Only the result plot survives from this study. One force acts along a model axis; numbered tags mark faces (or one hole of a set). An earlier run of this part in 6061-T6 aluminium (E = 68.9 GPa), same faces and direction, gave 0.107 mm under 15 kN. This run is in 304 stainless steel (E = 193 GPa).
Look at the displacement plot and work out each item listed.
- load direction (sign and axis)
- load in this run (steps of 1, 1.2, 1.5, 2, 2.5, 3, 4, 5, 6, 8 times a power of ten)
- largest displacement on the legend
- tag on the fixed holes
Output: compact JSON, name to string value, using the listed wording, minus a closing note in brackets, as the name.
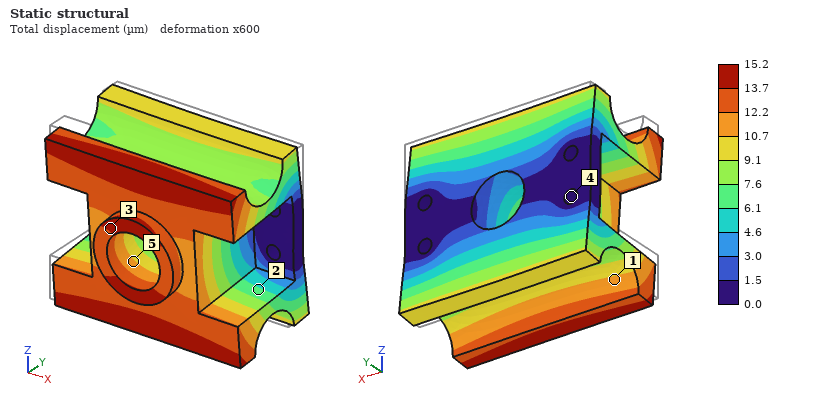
{"load direction": "-Z", "load in this run": "6 kN", "largest displacement on the legend": "15.2 µm", "tag on the fixed holes": "4"}
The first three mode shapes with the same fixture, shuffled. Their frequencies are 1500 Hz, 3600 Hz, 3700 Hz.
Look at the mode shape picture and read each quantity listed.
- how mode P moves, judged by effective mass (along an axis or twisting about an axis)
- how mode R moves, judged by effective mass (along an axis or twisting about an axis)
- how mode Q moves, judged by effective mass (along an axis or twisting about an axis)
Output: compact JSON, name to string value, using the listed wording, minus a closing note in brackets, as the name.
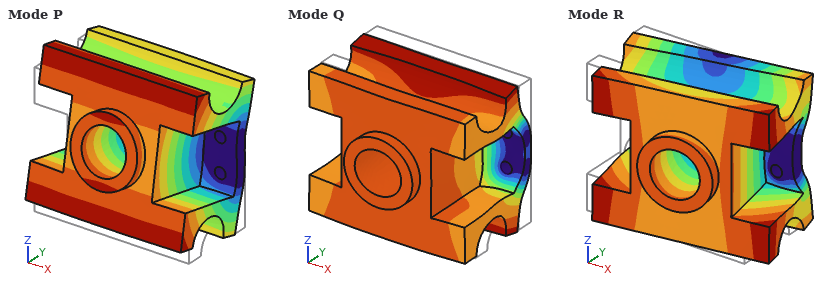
{"how mode P moves, judged by effective mass": "along Z", "how mode R moves, judged by effective mass": "along X", "how mode Q moves, judged by effective mass": "along Y"}
